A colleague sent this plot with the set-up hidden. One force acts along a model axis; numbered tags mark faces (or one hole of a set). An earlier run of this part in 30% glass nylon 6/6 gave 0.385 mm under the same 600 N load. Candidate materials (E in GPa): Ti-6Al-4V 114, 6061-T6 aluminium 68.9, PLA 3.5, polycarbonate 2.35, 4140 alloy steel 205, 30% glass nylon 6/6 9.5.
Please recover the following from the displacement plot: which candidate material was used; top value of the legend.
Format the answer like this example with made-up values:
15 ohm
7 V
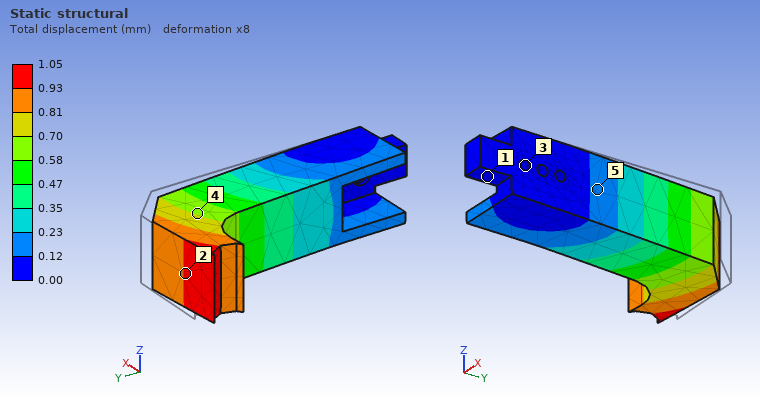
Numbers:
PLA
1.05 mm
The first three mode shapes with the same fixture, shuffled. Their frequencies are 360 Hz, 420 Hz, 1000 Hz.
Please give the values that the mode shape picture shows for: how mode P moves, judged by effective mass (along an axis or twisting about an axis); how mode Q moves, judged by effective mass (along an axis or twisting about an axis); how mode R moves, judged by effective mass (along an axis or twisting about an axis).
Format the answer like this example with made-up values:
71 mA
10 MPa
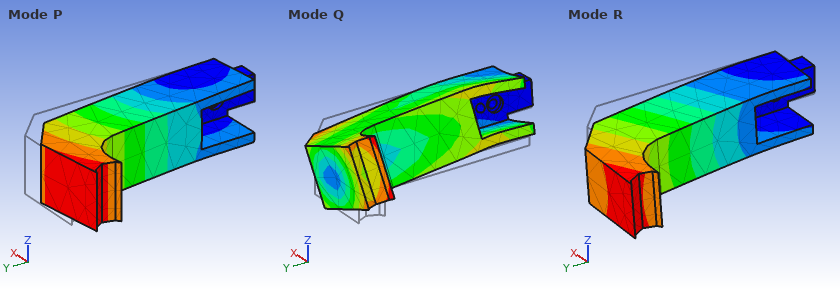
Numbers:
along X
twisting about Y
along Z
